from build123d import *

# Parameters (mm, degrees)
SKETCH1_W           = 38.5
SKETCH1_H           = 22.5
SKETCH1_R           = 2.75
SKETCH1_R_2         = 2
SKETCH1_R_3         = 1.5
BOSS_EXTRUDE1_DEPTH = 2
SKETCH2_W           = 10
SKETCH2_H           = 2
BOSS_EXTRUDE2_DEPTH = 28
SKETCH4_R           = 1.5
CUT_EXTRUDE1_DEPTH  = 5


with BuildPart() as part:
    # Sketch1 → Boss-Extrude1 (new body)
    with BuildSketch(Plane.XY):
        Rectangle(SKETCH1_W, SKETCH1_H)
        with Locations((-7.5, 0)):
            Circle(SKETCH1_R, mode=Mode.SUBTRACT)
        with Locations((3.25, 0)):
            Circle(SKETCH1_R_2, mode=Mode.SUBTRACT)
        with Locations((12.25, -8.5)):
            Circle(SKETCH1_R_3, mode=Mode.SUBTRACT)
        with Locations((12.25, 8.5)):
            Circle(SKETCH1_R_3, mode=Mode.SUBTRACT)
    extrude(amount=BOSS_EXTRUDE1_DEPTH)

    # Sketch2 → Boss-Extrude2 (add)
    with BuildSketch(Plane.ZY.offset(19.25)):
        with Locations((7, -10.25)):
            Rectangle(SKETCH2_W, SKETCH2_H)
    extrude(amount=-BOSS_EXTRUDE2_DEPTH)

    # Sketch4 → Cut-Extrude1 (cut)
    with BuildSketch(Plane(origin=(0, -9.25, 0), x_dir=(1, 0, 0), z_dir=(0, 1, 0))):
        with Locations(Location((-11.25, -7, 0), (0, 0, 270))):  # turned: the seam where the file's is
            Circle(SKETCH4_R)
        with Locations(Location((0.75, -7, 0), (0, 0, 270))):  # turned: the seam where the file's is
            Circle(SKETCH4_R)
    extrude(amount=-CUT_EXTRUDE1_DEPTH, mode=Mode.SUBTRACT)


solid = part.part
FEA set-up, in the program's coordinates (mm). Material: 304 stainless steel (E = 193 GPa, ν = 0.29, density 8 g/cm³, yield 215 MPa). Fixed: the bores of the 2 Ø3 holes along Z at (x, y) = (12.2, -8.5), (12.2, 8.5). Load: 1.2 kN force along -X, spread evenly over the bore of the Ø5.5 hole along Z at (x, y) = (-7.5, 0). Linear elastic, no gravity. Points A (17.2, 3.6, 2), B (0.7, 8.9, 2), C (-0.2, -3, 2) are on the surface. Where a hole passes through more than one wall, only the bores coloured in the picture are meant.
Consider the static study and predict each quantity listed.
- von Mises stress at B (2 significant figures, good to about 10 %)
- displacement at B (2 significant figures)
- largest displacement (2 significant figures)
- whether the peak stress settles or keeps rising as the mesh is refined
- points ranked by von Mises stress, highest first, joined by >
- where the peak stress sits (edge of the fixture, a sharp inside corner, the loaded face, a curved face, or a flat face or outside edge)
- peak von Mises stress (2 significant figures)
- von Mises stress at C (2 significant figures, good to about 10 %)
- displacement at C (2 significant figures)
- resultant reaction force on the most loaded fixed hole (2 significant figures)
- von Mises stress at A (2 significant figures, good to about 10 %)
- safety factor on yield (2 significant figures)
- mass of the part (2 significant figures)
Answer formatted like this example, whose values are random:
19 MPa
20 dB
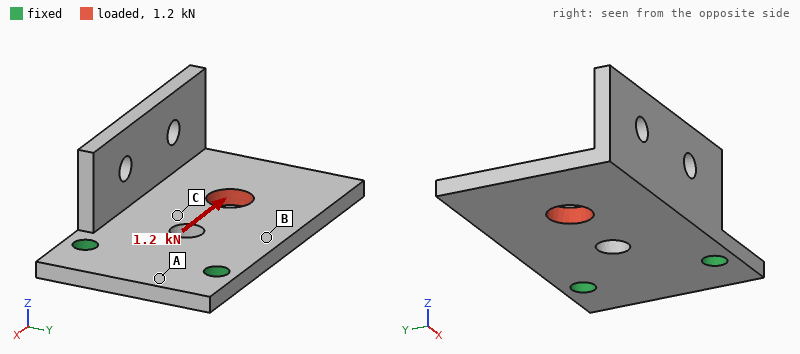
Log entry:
25 MPa
1.9 µm
5.5 µm
settles
C > B > A
a curved face
80 MPa
38 MPa
2.3 µm
600 N
8.8 MPa
2.7
17 g
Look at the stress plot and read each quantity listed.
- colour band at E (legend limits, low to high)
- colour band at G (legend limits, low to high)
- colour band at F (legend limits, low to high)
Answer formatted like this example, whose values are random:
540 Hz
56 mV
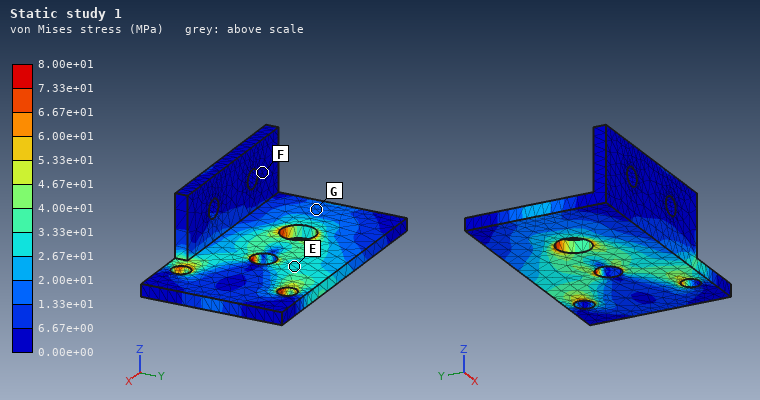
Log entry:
2.67e+01 to 3.33e+01 MPa
1.33e+01 to 2.00e+01 MPa
0.00e+00 to 6.67e+00 MPa
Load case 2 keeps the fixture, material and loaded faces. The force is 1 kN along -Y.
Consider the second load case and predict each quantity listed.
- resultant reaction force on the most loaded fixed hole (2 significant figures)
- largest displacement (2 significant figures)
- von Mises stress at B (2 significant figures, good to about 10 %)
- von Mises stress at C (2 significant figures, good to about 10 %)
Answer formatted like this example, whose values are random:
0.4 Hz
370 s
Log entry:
1.2 kN
23 µm
45 MPa
44 MPa
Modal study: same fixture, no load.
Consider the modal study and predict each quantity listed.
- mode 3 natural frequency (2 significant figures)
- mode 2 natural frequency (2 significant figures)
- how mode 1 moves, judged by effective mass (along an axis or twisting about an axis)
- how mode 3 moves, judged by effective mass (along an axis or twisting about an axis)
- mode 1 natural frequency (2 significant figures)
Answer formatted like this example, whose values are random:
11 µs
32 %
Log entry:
8300 Hz
3800 Hz
along Z
along Y
1500 Hz
